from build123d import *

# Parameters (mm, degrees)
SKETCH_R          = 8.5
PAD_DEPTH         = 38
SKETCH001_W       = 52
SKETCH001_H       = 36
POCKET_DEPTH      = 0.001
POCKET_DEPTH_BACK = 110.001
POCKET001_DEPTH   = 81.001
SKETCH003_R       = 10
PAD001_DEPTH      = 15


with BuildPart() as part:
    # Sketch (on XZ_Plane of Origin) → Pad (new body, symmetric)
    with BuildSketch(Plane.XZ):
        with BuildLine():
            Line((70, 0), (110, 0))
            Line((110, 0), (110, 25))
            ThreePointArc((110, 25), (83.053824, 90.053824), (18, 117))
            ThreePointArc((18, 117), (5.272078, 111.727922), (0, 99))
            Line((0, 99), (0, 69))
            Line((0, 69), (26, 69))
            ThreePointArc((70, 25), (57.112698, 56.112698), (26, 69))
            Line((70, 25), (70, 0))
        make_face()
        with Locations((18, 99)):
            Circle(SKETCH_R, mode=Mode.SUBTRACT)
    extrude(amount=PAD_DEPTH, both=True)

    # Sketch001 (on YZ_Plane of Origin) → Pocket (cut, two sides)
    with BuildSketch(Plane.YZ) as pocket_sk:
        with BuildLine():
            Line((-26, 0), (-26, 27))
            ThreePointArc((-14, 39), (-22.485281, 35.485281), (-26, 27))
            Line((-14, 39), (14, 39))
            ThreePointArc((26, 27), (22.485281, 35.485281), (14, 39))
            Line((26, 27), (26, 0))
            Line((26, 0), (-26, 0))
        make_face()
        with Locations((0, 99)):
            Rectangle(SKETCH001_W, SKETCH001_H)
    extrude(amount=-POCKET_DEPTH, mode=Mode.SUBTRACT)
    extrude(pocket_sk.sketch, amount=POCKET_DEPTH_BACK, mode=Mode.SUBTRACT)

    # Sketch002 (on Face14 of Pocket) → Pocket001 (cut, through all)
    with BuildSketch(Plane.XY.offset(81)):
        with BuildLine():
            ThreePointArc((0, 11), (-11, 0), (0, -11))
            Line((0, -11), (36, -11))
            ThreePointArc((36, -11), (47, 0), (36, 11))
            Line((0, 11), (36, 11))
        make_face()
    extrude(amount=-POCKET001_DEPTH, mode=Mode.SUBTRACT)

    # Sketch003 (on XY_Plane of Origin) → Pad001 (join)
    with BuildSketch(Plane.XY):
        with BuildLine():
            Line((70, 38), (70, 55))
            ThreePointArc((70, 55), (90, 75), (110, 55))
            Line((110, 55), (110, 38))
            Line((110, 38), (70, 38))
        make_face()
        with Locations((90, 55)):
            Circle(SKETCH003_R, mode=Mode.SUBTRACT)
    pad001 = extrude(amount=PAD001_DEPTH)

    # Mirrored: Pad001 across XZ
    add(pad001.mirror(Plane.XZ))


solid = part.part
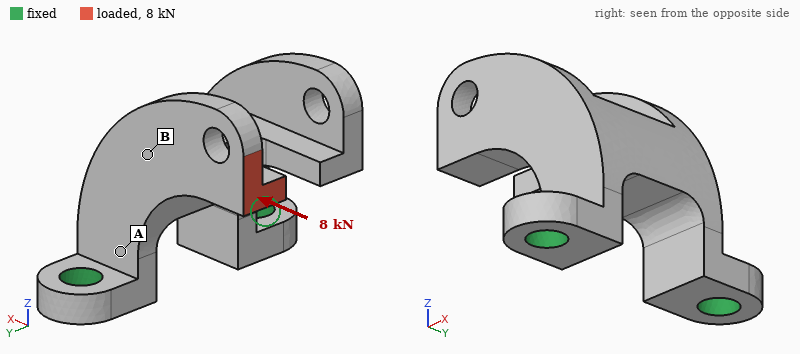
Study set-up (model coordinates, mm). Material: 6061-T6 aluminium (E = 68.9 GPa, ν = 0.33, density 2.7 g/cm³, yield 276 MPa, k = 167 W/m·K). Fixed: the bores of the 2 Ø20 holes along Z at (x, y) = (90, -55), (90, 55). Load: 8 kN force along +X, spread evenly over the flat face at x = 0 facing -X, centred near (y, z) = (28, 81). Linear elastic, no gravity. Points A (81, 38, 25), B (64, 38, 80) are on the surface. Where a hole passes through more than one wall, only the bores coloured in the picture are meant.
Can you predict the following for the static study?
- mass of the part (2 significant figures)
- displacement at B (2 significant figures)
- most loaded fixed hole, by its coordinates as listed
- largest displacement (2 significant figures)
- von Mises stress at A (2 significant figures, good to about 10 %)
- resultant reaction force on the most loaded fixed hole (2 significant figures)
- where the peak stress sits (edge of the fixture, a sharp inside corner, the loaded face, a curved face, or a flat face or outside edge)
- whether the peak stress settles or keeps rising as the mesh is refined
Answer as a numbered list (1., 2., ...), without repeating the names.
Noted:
1. 830 g
2. 0.42 mm
3. (90, 55)
4. 0.75 mm
5. 57 MPa
6. 6.6 kN
7. edge of the fixture
8. keeps rising
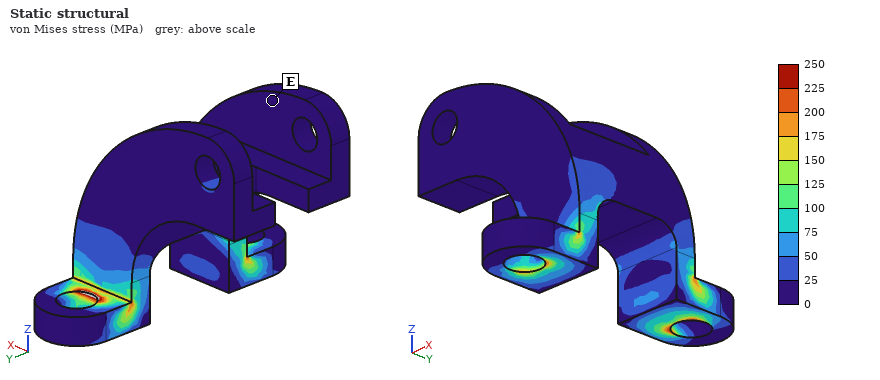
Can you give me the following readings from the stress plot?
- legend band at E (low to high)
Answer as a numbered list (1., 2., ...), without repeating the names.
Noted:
1. 0 to 25 MPa
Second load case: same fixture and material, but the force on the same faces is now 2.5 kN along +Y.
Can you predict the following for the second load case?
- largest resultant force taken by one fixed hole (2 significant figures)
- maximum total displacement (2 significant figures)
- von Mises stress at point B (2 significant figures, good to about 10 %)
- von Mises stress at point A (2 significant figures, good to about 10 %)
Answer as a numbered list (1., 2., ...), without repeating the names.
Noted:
1. 3.7 kN
2. 0.20 mm
3. 18 MPa
4. 30 MPa
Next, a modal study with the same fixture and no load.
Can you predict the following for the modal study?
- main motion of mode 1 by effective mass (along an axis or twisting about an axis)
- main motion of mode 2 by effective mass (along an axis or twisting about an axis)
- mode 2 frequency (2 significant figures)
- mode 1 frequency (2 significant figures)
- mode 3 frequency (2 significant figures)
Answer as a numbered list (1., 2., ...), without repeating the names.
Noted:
1. along X
2. along Y
3. 1800 Hz
4. 890 Hz
5. 3000 Hz
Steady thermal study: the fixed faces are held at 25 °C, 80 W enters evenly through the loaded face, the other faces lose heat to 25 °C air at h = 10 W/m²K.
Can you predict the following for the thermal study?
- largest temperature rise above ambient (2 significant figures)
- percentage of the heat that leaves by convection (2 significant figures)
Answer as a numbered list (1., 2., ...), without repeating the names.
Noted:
1. 73 K
2. 13 %
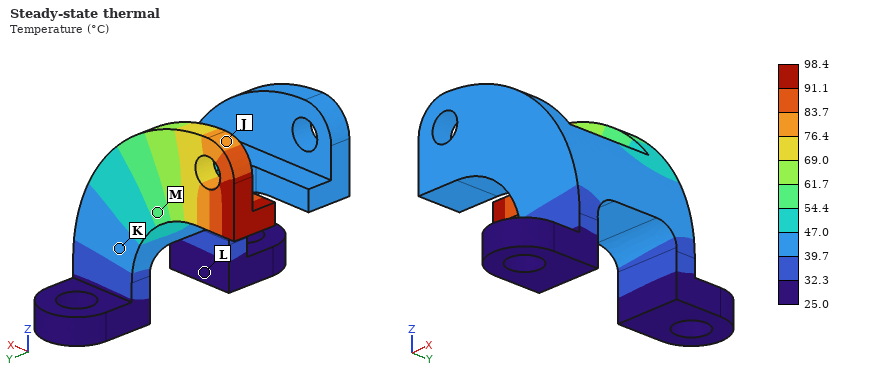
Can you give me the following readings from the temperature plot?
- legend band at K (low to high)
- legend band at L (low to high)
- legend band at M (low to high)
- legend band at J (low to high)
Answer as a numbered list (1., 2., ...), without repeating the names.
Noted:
1. 39.7 to 47.0 °C
2. 25.0 to 32.3 °C
3. 54.4 to 61.7 °C
4. 76.4 to 83.7 °C
